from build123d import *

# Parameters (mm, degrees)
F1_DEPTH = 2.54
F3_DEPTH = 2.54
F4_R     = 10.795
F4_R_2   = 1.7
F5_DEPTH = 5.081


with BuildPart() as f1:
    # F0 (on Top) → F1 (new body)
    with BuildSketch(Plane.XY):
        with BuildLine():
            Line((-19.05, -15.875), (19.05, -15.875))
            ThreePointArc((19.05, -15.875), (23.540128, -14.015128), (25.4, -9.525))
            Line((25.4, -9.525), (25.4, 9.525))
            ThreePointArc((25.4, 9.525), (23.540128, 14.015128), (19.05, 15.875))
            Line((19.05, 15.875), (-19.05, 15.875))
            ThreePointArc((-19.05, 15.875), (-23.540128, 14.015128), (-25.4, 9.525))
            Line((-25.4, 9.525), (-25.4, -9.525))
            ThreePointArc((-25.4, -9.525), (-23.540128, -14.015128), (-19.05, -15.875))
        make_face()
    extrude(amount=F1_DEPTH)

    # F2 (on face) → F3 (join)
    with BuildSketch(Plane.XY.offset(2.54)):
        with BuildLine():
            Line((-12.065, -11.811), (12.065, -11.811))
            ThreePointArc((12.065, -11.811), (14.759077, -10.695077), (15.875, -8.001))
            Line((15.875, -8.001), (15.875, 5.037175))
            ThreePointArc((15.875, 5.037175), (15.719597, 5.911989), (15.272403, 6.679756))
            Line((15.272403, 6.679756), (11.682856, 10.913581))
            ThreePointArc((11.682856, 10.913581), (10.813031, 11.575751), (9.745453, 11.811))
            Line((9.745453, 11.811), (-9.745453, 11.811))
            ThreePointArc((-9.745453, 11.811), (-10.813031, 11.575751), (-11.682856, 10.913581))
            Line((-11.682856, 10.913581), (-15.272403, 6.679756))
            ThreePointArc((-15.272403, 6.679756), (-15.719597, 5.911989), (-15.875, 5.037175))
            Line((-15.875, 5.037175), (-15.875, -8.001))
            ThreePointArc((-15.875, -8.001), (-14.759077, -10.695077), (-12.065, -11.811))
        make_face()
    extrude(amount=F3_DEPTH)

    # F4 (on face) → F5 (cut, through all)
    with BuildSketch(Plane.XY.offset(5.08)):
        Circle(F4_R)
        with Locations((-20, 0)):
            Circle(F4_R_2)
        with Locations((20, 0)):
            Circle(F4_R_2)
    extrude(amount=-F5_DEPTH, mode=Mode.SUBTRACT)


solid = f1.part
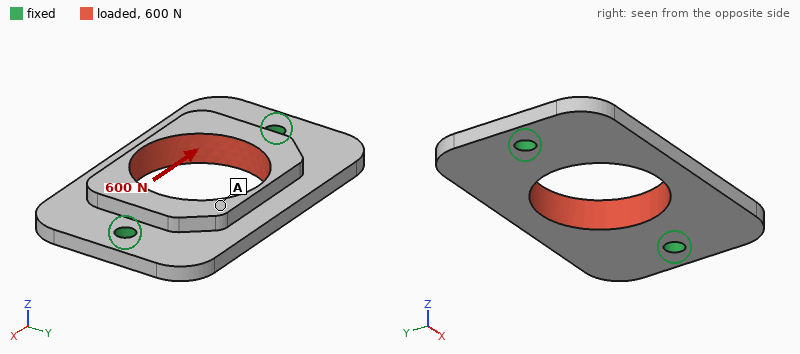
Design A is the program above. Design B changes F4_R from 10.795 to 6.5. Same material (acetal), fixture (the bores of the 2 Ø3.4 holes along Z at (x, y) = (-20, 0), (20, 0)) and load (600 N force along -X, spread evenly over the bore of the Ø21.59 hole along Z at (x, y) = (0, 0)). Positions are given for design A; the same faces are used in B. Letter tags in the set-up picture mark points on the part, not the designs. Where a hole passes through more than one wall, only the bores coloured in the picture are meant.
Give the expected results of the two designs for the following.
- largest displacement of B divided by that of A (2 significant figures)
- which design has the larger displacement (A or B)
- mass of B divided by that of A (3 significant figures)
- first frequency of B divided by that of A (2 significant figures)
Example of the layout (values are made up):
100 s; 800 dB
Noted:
0.68; A; 1.30; 0.97
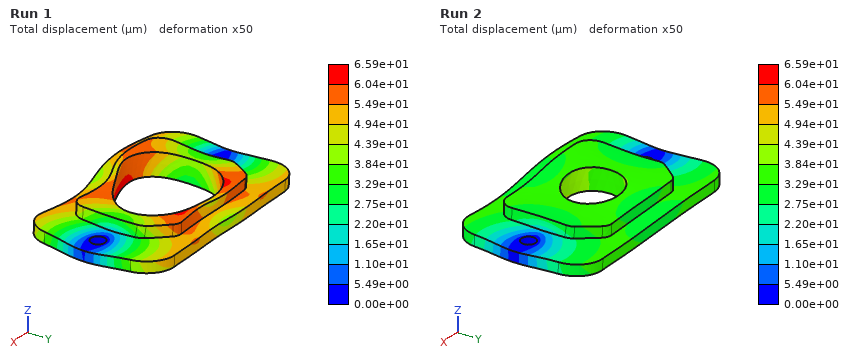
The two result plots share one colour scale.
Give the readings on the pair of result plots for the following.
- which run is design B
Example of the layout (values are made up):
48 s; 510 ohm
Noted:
Run 2
